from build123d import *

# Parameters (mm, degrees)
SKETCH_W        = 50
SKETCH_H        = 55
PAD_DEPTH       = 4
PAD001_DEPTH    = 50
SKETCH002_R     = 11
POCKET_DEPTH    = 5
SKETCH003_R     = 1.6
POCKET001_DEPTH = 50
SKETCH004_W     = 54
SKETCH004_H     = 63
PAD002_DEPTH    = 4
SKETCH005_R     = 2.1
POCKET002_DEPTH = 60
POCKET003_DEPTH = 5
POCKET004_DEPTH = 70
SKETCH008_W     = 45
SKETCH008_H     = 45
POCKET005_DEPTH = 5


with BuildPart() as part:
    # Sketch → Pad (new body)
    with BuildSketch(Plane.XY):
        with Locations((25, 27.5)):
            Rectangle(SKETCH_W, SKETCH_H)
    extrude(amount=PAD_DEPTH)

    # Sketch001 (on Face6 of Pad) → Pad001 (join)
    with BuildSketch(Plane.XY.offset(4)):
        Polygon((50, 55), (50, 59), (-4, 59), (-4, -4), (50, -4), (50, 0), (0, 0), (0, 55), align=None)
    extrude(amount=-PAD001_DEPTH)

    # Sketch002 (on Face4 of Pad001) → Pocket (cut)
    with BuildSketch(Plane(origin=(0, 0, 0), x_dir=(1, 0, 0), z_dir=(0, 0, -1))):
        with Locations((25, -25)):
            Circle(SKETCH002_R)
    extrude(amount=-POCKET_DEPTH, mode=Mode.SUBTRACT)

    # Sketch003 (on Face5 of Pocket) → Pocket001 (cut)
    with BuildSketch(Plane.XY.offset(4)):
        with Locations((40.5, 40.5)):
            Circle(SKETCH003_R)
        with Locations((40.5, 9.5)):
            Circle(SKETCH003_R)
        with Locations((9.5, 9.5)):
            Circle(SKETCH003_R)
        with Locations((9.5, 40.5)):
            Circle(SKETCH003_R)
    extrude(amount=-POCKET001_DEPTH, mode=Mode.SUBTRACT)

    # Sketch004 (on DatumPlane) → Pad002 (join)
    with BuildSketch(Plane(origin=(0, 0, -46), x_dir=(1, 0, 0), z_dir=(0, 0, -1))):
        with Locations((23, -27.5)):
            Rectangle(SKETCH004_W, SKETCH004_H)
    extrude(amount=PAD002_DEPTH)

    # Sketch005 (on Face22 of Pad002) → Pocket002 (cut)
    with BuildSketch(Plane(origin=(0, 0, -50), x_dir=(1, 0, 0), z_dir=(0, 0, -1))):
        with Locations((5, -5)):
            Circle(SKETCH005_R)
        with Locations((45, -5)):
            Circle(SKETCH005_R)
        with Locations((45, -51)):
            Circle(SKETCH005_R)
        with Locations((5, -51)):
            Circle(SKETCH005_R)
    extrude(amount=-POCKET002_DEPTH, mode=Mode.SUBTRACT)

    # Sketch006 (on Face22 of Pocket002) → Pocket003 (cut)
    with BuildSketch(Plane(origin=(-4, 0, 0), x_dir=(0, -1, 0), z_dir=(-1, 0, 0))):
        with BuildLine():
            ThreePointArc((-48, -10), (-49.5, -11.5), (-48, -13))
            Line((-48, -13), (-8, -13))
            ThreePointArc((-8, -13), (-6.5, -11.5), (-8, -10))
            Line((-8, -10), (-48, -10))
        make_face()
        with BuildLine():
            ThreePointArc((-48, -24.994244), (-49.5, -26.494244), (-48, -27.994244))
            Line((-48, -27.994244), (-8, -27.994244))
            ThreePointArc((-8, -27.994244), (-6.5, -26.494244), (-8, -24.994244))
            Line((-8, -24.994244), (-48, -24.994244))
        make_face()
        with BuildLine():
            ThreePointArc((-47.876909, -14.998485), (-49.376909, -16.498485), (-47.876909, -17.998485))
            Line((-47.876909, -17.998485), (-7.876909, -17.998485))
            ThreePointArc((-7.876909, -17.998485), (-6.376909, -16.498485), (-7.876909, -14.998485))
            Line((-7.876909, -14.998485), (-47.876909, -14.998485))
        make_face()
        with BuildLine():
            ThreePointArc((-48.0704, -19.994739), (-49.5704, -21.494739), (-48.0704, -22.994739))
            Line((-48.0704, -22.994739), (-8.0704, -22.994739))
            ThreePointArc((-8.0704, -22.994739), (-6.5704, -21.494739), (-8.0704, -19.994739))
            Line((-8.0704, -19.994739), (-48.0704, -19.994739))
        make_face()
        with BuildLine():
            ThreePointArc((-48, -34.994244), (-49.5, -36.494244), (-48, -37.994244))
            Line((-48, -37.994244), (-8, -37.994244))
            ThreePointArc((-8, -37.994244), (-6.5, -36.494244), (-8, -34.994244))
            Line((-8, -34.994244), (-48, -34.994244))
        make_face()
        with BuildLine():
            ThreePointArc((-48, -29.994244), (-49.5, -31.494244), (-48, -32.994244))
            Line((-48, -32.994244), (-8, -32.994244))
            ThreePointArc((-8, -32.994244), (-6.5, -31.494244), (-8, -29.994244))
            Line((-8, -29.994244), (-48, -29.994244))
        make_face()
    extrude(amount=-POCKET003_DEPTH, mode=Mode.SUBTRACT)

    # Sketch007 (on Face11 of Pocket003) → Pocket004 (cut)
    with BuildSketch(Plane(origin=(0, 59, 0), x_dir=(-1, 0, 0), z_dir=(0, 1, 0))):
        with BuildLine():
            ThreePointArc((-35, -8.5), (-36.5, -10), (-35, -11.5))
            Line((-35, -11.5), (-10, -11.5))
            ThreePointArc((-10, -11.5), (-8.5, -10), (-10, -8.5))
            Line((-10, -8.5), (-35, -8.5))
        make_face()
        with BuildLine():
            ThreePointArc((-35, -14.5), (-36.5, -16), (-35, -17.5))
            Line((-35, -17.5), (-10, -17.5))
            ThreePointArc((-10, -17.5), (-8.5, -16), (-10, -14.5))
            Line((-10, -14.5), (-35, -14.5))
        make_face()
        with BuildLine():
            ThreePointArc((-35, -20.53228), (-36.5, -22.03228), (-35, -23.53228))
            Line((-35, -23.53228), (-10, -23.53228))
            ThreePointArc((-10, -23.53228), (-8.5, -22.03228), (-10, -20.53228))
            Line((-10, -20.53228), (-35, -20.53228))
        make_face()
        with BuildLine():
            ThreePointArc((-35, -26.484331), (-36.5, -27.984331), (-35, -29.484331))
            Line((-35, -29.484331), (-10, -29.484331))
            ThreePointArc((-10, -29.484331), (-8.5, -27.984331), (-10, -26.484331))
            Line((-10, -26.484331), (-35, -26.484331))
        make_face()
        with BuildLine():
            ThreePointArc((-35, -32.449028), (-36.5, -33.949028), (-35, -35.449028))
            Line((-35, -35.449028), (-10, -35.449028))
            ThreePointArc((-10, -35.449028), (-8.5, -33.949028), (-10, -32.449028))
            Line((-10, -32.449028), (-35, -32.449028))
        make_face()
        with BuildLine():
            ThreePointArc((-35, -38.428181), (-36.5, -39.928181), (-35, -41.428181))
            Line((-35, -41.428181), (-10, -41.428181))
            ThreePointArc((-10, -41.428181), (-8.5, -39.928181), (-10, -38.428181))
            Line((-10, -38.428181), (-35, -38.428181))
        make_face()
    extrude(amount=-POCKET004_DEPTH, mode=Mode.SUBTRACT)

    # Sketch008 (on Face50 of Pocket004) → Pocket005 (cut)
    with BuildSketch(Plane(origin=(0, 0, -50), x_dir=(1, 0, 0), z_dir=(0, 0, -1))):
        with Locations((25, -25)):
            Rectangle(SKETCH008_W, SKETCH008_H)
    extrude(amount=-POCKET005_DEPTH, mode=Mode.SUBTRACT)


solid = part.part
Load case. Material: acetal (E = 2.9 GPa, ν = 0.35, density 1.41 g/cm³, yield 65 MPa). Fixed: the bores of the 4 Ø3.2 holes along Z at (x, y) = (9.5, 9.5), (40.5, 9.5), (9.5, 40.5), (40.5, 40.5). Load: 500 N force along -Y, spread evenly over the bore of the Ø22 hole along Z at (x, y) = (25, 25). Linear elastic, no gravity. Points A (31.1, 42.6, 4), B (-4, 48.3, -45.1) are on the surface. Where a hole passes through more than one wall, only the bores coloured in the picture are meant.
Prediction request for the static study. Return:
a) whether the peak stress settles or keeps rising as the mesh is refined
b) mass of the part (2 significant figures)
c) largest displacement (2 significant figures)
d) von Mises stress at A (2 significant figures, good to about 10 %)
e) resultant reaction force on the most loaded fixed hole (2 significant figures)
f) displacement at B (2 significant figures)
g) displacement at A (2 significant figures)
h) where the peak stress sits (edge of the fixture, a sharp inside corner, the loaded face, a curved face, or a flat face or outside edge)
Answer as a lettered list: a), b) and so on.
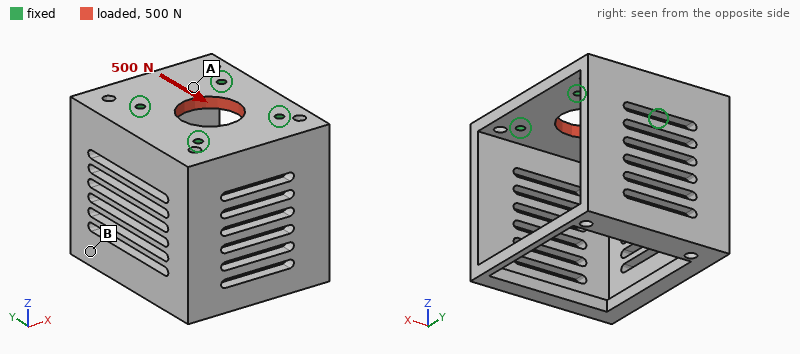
a) keeps rising
b) 57 g
c) 17 µm
d) 1.3 MPa
e) 130 N
f) 3.2 µm
g) 10 µm
h) edge of the fixture
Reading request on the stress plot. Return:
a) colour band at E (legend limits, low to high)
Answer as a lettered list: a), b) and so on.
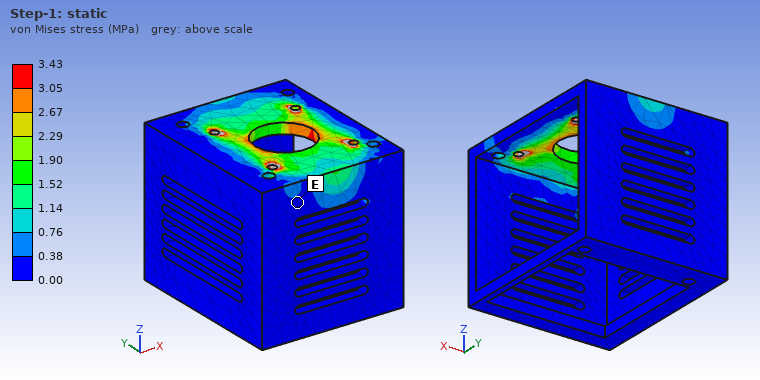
a) 0.00 to 0.38 MPa
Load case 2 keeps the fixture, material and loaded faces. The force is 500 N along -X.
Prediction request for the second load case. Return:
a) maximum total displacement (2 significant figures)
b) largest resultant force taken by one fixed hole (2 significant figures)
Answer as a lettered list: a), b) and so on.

a) 21 µm
b) 130 N
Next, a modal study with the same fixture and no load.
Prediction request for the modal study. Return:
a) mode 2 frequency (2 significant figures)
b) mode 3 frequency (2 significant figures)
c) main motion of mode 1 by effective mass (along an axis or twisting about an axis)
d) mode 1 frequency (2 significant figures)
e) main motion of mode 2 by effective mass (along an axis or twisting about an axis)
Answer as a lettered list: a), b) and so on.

a) 530 Hz
b) 780 Hz
c) along Y
d) 380 Hz
e) along X
